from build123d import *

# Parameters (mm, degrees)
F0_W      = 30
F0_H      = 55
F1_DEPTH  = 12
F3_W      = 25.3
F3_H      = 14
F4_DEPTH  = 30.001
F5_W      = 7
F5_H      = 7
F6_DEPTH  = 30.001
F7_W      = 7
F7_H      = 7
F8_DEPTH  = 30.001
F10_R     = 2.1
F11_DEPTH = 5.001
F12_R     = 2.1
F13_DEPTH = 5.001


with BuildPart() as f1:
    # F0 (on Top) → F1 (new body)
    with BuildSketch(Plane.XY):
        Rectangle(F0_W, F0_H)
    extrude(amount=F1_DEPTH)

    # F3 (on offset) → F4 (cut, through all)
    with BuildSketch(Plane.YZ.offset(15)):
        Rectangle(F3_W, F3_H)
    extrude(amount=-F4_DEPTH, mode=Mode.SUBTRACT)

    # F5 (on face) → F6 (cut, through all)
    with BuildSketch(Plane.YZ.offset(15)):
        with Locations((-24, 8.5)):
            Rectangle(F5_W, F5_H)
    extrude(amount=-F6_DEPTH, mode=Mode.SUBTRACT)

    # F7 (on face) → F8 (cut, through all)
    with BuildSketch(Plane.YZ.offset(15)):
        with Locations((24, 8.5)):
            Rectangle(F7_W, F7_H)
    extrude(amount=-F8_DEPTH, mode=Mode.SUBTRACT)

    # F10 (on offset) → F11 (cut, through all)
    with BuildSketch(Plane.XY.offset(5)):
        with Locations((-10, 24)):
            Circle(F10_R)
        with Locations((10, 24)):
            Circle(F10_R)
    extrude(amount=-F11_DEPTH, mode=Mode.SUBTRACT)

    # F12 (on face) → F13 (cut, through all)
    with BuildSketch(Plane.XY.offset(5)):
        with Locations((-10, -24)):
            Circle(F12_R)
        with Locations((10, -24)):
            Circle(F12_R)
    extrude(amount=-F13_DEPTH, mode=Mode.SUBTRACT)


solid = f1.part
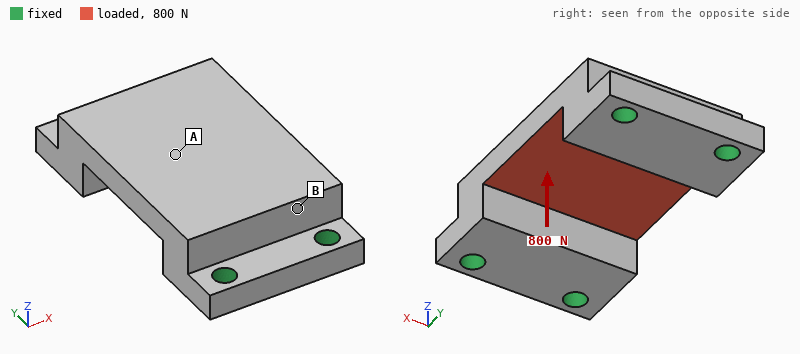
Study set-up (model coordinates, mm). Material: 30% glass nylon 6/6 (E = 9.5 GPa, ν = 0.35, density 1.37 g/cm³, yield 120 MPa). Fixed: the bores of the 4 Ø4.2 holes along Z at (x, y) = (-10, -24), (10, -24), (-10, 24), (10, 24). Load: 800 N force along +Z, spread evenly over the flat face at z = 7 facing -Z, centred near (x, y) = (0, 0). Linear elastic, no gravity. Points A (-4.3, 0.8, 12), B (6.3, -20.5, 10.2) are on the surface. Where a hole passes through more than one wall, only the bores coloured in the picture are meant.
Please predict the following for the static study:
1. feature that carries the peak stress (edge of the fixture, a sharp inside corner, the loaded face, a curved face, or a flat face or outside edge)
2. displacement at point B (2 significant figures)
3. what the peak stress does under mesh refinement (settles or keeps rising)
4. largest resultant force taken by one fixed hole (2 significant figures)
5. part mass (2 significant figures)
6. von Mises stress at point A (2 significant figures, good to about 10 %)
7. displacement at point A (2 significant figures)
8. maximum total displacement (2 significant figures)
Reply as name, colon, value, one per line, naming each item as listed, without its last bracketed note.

feature that carries the peak stress: edge of the fixture
displacement at point B: 8.9 µm
what the peak stress does under mesh refinement: keeps rising
largest resultant force taken by one fixed hole: 350 N
part mass: 15 g
von Mises stress at point A: 14 MPa
displacement at point A: 48 µm
maximum total displacement: 54 µm
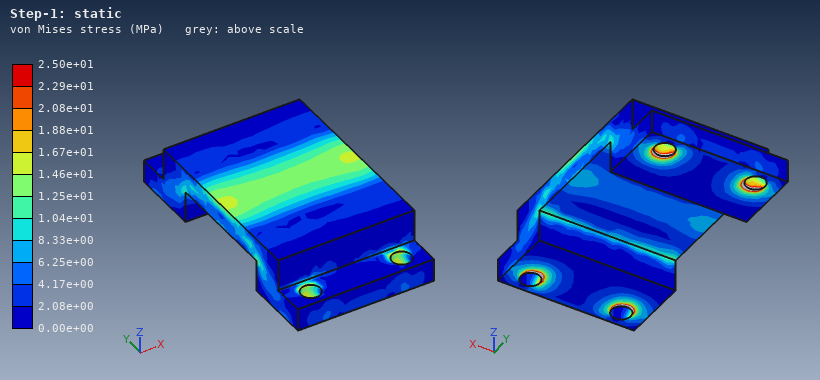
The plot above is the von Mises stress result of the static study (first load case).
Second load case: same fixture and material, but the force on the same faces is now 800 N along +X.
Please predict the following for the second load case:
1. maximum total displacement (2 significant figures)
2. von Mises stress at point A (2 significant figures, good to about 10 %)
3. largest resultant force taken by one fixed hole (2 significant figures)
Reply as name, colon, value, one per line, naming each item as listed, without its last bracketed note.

maximum total displacement: 25 µm
von Mises stress at point A: 1.5 MPa
largest resultant force taken by one fixed hole: 260 N
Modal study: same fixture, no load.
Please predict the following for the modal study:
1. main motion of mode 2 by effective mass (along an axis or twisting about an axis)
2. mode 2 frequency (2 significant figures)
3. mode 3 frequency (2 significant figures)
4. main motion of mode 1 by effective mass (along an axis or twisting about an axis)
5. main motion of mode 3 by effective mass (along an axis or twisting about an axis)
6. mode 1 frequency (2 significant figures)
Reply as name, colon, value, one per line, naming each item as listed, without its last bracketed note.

main motion of mode 2 by effective mass: along Y
mode 2 frequency: 9700 Hz
mode 3 frequency: 10 kHz
main motion of mode 1 by effective mass: along Z
main motion of mode 3 by effective mass: along X
mode 1 frequency: 8900 Hz
